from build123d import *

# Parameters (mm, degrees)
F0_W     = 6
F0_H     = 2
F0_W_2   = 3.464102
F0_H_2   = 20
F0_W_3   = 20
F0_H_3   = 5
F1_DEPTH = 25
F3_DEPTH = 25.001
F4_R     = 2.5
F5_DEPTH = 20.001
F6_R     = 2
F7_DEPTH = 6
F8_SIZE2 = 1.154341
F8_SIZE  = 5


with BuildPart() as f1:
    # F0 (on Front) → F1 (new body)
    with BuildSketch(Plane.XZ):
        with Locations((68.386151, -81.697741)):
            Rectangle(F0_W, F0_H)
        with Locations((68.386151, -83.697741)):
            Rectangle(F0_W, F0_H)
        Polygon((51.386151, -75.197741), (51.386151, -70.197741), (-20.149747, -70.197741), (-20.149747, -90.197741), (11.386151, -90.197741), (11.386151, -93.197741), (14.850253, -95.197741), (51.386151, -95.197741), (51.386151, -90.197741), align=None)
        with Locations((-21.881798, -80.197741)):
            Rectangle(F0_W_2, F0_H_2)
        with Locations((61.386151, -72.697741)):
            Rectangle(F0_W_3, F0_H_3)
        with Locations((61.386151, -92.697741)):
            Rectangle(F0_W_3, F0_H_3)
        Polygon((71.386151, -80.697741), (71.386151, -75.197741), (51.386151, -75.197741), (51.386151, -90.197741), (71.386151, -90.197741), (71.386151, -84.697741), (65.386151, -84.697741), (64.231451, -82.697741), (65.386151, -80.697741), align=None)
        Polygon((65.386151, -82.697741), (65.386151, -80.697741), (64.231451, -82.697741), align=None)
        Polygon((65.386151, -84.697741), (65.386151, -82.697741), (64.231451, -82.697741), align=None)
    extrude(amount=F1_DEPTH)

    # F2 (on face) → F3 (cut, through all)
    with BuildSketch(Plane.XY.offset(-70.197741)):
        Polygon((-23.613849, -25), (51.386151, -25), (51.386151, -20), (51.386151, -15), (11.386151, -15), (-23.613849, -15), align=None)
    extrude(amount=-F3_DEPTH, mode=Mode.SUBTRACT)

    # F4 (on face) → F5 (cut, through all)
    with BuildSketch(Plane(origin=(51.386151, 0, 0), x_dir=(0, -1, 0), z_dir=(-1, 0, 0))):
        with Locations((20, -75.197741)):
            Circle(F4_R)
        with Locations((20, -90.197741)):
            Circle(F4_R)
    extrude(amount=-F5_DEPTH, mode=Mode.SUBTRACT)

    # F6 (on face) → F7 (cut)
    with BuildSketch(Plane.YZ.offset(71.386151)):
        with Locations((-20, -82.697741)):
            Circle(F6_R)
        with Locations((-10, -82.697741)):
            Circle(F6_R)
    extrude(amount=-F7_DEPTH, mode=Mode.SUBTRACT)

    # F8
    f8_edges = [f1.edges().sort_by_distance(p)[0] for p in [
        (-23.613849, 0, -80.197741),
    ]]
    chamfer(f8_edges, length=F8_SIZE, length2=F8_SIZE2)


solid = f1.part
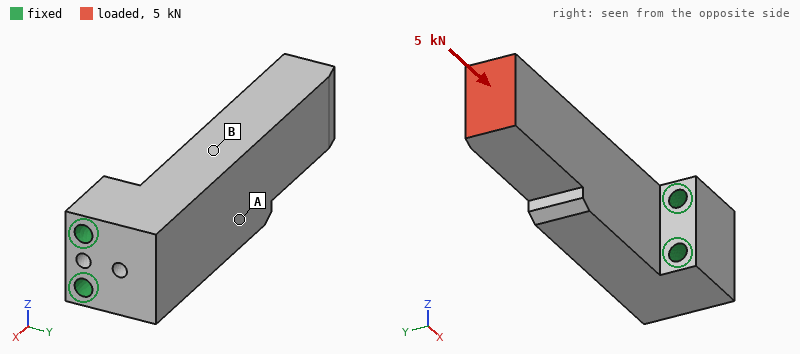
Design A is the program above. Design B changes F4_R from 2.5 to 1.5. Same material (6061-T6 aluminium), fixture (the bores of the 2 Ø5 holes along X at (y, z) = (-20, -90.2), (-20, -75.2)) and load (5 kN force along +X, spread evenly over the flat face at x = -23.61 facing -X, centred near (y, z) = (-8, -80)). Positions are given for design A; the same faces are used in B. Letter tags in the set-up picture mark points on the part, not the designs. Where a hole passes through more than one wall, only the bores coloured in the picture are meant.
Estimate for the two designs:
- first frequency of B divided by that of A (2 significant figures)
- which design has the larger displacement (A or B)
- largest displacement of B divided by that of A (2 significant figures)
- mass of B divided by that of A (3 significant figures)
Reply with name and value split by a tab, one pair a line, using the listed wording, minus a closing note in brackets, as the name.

first frequency of B divided by that of A	0.98
which design has the larger displacement	B
largest displacement of B divided by that of A	1.1
mass of B divided by that of A	1.01
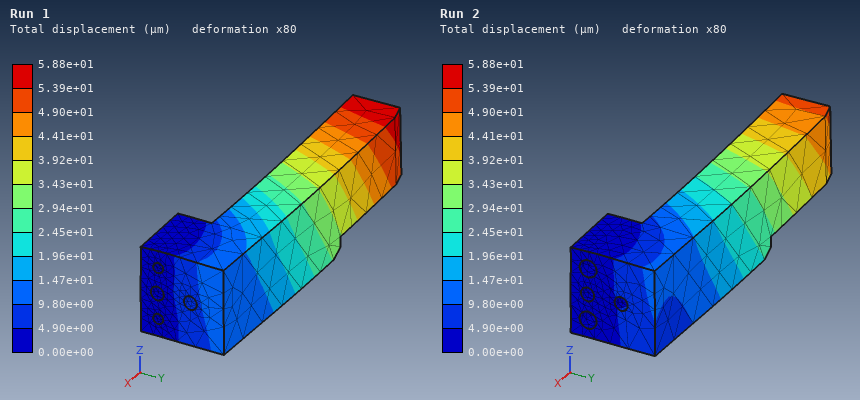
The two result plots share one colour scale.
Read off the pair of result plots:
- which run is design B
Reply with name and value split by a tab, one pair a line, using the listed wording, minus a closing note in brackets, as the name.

which run is design B	Run 1
